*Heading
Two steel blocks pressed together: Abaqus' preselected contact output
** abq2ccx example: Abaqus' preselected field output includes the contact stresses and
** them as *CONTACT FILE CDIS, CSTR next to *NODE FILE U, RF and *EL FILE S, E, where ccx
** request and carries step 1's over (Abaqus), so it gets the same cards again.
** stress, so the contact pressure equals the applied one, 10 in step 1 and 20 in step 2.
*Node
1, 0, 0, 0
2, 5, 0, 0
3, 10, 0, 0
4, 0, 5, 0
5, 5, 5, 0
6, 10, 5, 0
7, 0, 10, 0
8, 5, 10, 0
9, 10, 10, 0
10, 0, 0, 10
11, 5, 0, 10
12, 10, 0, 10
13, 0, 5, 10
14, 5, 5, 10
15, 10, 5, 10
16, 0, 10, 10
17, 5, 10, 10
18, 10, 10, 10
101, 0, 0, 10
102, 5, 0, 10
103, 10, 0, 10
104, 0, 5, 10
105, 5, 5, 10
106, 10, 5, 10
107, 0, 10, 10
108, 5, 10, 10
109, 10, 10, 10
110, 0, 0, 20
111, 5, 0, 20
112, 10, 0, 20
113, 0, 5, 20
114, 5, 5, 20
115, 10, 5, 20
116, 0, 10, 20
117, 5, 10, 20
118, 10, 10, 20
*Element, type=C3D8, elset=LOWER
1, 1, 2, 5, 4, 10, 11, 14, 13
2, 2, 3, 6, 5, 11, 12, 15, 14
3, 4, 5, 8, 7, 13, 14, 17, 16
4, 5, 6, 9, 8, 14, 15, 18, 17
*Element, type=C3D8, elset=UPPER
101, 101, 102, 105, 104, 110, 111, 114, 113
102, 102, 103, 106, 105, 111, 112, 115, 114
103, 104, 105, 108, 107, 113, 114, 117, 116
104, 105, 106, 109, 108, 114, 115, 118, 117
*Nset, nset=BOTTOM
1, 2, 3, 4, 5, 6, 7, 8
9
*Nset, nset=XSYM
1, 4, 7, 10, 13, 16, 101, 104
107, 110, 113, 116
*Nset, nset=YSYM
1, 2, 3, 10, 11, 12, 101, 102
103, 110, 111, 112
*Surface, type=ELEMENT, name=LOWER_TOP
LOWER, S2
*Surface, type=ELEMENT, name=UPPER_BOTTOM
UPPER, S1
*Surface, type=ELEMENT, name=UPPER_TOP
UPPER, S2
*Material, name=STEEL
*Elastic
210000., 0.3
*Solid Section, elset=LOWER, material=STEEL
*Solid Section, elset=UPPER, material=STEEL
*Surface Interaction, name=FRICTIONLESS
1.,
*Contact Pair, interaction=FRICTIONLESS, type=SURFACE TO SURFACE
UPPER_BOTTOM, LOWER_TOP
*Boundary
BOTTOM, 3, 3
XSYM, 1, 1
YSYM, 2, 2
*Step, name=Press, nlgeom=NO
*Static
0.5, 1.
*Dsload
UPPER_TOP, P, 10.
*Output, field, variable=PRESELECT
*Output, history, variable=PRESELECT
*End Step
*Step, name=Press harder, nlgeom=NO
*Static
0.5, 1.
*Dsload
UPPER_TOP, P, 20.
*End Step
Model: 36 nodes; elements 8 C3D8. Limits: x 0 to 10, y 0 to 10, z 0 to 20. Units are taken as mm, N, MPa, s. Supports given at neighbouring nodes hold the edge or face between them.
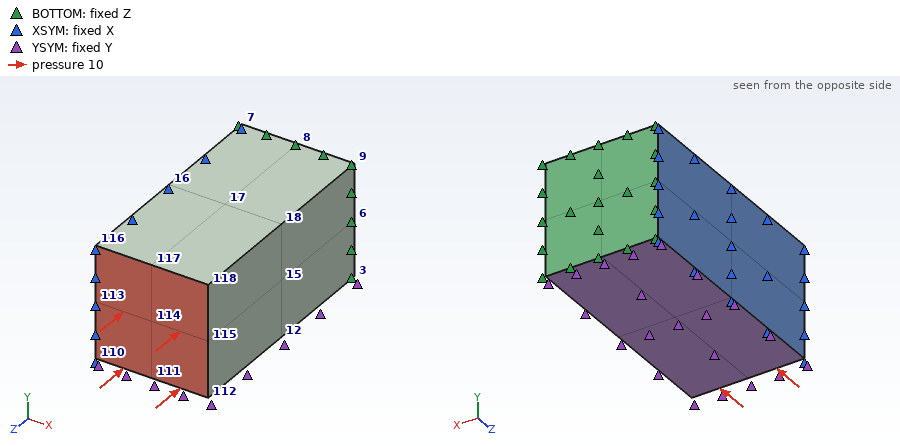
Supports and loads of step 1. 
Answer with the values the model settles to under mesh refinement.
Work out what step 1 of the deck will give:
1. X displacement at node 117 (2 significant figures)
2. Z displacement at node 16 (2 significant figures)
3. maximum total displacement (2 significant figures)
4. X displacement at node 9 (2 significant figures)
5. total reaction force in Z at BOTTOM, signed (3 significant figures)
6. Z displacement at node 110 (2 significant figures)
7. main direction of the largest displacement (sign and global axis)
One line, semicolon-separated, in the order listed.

7.1e-05 mm; -4.8e-04 mm; 9.7e-04 mm; 1.4e-04 mm; 1000 N; -9.5e-04 mm; -Z
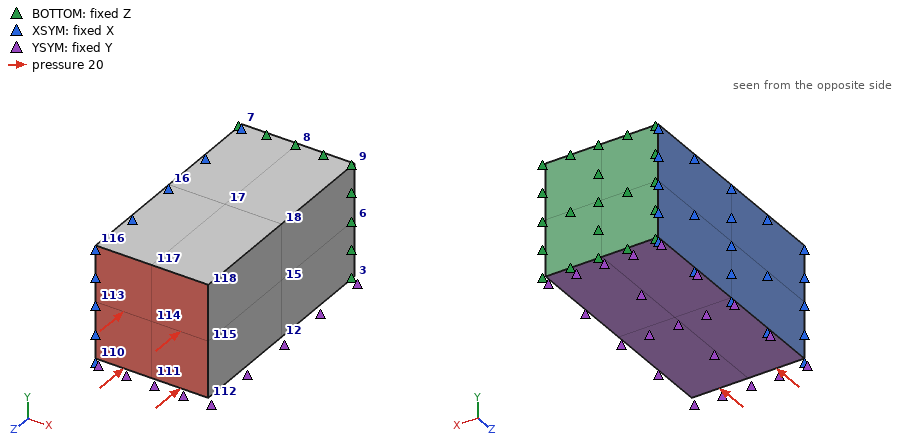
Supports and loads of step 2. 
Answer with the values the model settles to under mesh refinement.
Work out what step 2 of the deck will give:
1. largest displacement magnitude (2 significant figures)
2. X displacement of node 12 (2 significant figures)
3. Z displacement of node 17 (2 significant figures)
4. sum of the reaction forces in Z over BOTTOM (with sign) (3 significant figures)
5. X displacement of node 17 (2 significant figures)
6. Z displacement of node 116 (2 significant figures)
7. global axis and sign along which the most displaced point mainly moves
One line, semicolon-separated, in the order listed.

0.0019 mm; 2.9e-04 mm; -9.5e-04 mm; 2000 N; 1.4e-04 mm; -0.0019 mm; -Z
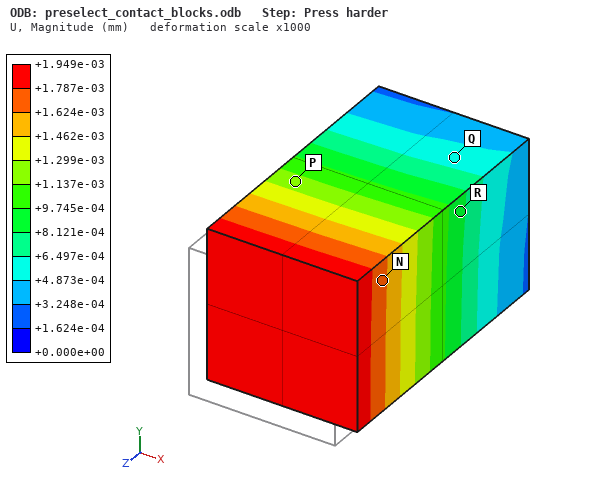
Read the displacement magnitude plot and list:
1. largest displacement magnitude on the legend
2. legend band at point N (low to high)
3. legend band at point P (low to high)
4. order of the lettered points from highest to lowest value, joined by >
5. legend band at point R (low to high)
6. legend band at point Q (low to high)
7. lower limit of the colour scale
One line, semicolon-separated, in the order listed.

+1.949e-03 mm; +1.624e-03 to +1.787e-03 mm; +1.137e-03 to +1.299e-03 mm; N > P > R > Q; +8.121e-04 to +9.745e-04 mm; +4.873e-04 to +6.497e-04 mm; +0.000e+00 mm
